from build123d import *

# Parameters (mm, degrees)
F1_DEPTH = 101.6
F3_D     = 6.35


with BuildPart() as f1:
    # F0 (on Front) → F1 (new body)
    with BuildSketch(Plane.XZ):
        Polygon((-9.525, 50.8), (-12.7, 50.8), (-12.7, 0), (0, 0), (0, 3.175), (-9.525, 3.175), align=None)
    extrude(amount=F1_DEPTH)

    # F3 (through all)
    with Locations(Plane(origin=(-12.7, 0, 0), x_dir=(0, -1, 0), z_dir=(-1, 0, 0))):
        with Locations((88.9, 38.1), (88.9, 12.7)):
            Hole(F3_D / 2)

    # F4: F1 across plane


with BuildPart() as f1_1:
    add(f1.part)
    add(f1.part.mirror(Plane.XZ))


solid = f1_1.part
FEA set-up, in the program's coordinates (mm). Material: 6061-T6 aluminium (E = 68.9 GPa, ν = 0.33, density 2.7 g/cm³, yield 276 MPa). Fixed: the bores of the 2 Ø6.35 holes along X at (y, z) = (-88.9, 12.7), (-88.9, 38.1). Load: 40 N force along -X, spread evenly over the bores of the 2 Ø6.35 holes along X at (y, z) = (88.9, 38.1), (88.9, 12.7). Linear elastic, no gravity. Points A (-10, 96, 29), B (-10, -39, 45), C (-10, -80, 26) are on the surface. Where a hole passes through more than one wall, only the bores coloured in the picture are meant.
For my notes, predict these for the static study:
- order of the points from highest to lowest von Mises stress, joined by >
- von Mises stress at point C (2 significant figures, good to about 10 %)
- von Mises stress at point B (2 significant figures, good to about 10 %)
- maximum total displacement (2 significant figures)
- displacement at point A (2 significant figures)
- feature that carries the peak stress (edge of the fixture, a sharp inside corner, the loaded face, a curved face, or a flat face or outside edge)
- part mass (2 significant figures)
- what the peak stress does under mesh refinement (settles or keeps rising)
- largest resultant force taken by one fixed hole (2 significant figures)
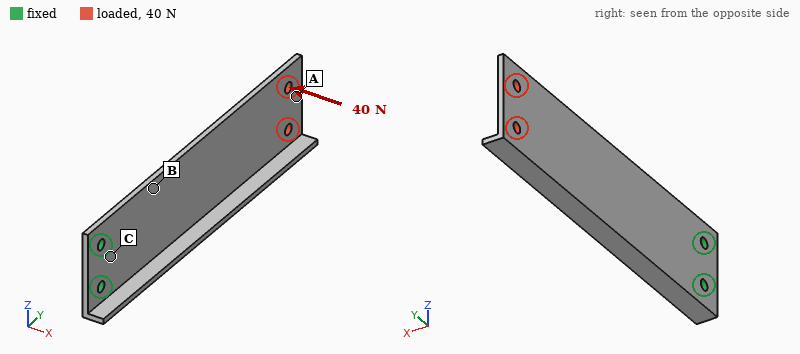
C > B > A
29 MPa
16 MPa
2.1 mm
1.9 mm
edge of the fixture
100 g
keeps rising
56 N
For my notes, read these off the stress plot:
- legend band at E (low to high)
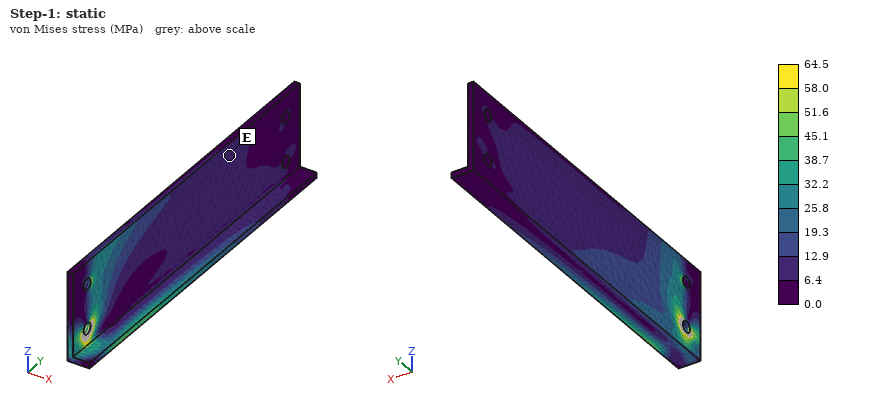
6.4 to 12.9 MPa
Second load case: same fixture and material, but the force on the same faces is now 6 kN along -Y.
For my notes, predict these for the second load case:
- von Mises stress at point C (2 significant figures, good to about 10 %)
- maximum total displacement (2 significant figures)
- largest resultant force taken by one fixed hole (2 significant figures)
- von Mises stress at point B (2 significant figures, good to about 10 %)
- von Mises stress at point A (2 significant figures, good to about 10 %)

23 MPa
0.88 mm
3.0 kN
33 MPa
16 MPa
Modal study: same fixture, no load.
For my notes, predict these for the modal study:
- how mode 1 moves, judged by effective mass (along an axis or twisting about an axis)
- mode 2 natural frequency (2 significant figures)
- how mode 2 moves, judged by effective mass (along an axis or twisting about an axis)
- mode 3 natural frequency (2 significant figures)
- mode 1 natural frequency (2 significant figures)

along X
490 Hz
twisting about Y
830 Hz
140 Hz
